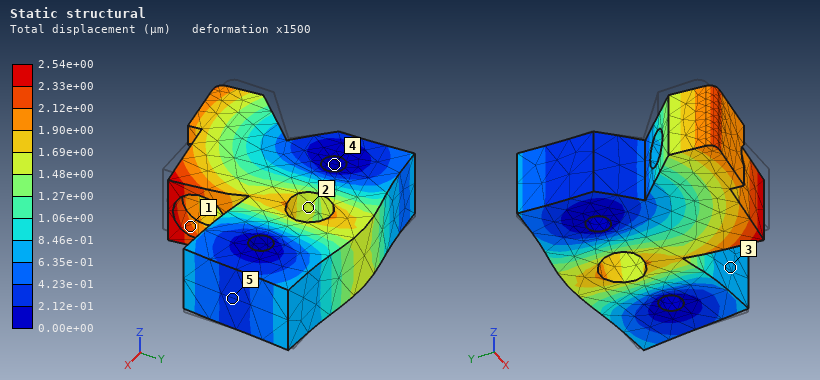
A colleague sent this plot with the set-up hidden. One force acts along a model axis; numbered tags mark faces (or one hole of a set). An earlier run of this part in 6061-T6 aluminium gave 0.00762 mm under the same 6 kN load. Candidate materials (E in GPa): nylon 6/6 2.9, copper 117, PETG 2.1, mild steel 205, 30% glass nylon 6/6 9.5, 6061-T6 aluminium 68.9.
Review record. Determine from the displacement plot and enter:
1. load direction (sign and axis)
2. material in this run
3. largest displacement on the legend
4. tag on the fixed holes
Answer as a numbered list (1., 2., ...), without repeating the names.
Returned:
1. +Y
2. mild steel
3. 2.54e+00 µm
4. 4
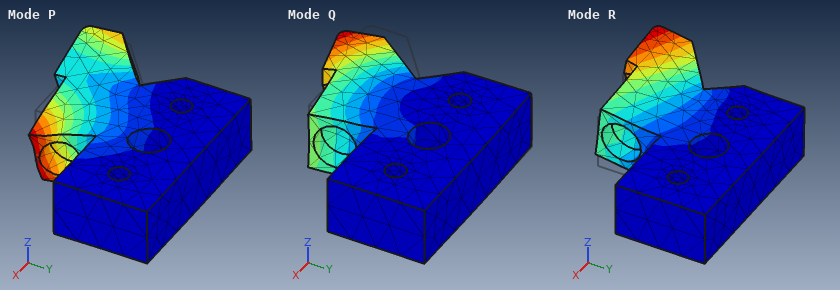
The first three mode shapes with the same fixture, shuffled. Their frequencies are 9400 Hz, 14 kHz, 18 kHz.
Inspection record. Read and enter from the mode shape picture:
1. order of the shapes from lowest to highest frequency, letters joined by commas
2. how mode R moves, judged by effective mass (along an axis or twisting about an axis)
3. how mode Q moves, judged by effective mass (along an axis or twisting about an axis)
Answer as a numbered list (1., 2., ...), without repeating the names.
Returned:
1. R, Q, P
2. along Z
3. along X
